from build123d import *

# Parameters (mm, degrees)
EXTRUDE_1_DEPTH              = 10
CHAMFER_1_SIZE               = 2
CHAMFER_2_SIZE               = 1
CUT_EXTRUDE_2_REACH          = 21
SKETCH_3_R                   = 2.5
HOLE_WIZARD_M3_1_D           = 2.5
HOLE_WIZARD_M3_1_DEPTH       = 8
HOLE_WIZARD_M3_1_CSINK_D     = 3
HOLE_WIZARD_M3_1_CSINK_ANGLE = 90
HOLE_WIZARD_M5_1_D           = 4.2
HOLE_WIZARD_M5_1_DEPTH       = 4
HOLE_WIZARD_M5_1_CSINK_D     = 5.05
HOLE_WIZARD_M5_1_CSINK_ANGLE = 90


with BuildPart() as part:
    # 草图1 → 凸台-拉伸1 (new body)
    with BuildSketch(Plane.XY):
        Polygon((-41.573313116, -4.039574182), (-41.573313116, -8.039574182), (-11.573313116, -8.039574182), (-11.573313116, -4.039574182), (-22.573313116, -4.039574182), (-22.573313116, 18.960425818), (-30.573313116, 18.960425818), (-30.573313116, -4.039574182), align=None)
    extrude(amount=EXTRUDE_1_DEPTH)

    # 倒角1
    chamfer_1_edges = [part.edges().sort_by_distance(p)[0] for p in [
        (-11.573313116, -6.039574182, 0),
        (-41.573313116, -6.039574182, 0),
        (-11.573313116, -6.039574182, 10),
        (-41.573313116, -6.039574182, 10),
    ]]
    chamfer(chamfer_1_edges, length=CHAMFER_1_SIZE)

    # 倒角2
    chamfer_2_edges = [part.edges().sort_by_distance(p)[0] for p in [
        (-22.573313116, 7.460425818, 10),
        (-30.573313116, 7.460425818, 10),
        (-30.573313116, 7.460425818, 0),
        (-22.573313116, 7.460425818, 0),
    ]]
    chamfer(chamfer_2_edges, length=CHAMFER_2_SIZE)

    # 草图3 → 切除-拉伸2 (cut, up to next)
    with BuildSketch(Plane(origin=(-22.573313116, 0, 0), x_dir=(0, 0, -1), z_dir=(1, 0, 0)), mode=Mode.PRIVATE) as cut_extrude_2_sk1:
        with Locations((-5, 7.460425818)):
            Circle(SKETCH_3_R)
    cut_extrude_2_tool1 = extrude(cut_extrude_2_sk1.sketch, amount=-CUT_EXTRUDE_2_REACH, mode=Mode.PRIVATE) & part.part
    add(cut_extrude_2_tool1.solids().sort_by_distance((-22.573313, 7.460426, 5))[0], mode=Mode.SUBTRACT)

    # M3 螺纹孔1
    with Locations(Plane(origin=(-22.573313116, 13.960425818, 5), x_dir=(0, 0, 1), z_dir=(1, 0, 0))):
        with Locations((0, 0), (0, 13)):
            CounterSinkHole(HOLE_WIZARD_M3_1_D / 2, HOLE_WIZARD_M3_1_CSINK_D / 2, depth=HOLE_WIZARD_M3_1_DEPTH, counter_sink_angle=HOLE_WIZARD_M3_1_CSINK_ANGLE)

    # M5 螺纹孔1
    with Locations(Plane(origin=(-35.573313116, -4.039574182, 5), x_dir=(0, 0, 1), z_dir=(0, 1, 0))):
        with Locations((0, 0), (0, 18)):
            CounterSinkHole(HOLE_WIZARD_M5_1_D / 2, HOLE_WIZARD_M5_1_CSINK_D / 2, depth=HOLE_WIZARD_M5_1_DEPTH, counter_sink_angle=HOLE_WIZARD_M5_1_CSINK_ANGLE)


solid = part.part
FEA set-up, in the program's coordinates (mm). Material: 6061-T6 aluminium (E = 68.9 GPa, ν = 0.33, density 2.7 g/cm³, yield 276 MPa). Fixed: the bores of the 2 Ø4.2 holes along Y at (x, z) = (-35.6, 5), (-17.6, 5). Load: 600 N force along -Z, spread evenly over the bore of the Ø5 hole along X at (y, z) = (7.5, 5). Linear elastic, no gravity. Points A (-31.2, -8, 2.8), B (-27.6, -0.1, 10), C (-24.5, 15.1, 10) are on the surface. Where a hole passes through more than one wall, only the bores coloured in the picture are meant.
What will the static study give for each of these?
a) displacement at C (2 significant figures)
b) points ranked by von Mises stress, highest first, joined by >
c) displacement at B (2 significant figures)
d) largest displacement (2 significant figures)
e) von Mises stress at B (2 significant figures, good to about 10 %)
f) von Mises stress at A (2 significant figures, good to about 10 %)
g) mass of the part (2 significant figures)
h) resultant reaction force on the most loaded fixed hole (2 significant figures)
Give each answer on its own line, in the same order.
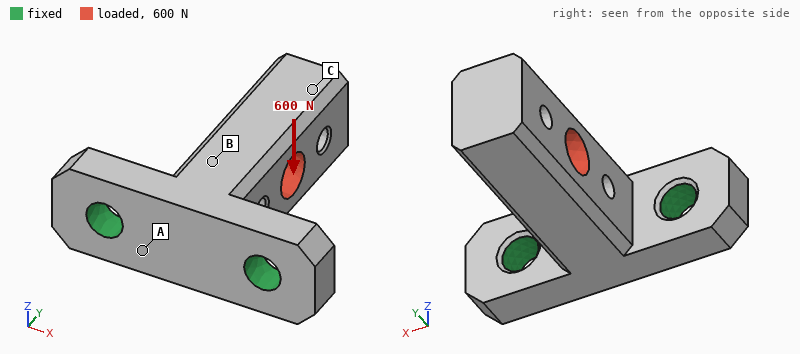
0.11 mm
A > B > C
0.036 mm
0.13 mm
40 MPa
67 MPa
7.1 g
300 N
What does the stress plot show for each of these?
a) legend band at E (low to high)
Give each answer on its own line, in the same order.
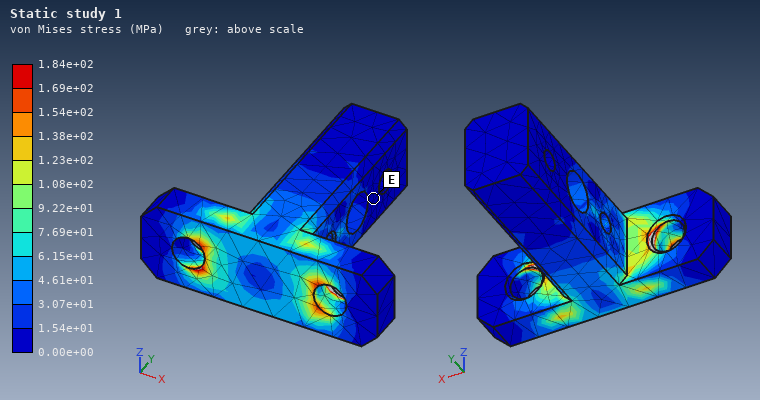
0.00e+00 to 1.54e+01 MPa
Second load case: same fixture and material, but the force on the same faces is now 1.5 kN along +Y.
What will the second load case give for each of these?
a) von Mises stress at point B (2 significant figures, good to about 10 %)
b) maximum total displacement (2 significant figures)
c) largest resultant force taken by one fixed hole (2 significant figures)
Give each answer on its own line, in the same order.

18 MPa
13 µm
790 N
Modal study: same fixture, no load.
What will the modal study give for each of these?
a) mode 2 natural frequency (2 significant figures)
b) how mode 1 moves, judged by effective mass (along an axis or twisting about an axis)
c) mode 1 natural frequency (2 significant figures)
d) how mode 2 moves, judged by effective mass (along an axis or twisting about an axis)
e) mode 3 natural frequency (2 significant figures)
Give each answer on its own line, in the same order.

8300 Hz
along Z
6200 Hz
along X
25 kHz
